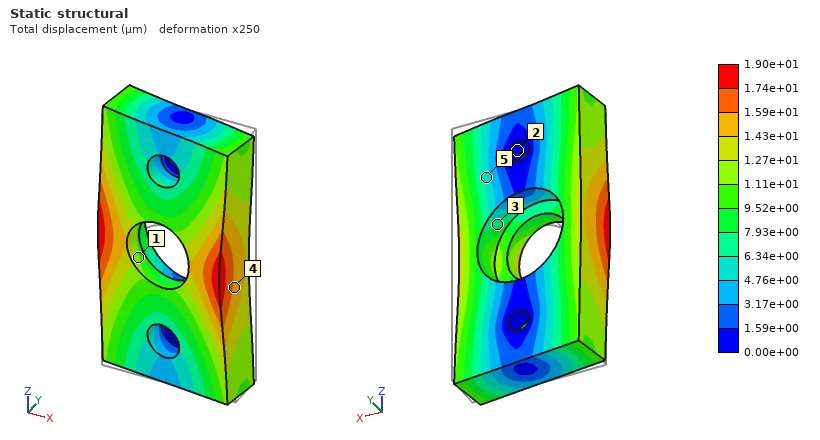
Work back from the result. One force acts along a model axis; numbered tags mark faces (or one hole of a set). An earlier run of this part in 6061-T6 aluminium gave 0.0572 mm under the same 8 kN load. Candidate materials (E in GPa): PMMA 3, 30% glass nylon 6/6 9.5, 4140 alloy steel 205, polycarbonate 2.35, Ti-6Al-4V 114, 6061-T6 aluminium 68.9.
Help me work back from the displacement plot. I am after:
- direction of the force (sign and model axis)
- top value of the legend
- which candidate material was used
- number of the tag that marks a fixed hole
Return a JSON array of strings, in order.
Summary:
["-X", "1.90e+01 µm", "4140 alloy steel", "2"]
